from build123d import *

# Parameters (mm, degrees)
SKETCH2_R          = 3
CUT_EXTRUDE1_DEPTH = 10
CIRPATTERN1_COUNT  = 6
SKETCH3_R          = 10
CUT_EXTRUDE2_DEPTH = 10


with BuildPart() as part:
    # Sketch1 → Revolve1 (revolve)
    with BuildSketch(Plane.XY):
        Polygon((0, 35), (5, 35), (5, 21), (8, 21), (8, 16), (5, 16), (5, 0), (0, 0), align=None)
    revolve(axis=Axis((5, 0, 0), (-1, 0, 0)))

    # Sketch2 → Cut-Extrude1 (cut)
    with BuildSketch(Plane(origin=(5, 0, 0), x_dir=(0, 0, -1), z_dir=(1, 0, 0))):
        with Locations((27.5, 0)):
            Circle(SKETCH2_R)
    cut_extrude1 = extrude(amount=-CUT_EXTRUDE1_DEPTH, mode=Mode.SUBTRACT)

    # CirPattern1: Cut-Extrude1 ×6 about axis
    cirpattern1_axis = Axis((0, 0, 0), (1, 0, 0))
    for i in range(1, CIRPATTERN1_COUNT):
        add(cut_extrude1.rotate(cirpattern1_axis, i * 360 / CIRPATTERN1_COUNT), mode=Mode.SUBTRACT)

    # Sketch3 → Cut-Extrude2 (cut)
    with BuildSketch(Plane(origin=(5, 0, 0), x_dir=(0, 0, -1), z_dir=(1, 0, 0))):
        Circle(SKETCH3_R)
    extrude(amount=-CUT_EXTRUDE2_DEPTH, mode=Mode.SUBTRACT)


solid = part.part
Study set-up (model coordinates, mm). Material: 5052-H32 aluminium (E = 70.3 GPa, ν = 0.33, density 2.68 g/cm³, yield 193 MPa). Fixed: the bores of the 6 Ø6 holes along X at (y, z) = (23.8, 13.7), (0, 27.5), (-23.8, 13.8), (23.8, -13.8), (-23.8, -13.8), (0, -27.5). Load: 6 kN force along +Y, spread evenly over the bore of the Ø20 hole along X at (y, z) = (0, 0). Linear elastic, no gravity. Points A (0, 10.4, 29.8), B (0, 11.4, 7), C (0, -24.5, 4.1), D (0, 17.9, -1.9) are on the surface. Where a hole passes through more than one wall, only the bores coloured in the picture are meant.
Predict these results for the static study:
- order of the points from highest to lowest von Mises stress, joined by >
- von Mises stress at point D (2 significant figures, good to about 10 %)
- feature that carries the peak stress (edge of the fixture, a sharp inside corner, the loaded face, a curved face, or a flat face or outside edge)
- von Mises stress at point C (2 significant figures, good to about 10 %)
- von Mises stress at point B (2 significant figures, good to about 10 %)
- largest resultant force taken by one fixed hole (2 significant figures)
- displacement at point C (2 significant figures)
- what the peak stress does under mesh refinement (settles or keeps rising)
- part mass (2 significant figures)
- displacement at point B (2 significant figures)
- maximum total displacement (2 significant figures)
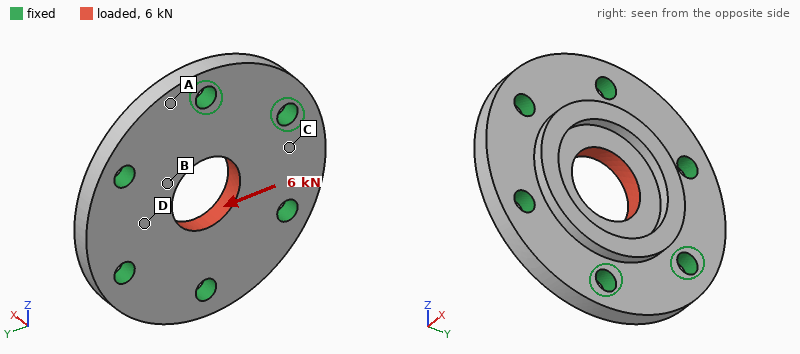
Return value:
B > D > C > A
13 MPa
edge of the fixture
6.8 MPa
19 MPa
1.3 kN
2.1 µm
keeps rising
50 g
3.6 µm
5.0 µm
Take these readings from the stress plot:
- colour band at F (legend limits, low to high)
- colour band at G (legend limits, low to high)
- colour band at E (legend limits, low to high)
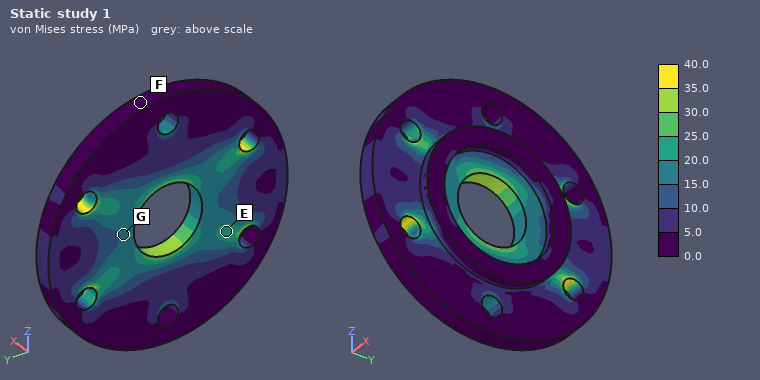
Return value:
0.0 to 5.0 MPa
15.0 to 20.0 MPa
20.0 to 25.0 MPa
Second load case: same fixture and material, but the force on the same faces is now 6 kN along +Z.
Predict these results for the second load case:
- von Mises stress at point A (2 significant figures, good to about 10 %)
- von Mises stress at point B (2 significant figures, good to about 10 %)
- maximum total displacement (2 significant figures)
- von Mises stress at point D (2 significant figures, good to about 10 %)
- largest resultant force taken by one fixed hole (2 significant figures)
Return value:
4.9 MPa
15 MPa
5.0 µm
9.4 MPa
1.5 kN
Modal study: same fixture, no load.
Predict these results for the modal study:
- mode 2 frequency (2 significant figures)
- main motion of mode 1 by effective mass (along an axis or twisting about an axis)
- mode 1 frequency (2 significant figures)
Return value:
27 kHz
along X
19 kHz
